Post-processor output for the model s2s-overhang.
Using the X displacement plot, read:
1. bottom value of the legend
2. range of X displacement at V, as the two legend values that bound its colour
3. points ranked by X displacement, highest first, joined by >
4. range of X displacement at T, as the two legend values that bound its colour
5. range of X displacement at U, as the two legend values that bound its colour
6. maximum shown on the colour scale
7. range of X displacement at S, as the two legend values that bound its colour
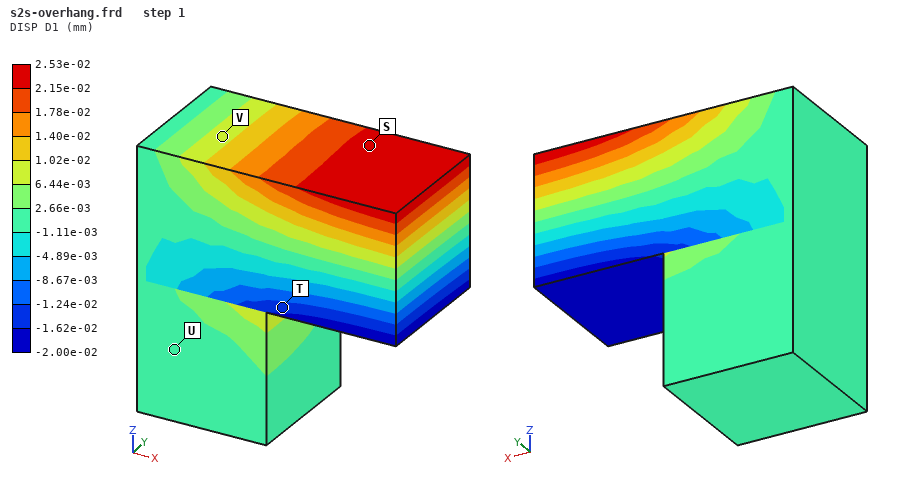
-2.00e-02 mm
6.44e-03 to 1.02e-02 mm
S > V > U > T
-1.62e-02 to -1.24e-02 mm
-1.11e-03 to 2.66e-03 mm
2.53e-02 mm
2.15e-02 to 2.53e-02 mm
